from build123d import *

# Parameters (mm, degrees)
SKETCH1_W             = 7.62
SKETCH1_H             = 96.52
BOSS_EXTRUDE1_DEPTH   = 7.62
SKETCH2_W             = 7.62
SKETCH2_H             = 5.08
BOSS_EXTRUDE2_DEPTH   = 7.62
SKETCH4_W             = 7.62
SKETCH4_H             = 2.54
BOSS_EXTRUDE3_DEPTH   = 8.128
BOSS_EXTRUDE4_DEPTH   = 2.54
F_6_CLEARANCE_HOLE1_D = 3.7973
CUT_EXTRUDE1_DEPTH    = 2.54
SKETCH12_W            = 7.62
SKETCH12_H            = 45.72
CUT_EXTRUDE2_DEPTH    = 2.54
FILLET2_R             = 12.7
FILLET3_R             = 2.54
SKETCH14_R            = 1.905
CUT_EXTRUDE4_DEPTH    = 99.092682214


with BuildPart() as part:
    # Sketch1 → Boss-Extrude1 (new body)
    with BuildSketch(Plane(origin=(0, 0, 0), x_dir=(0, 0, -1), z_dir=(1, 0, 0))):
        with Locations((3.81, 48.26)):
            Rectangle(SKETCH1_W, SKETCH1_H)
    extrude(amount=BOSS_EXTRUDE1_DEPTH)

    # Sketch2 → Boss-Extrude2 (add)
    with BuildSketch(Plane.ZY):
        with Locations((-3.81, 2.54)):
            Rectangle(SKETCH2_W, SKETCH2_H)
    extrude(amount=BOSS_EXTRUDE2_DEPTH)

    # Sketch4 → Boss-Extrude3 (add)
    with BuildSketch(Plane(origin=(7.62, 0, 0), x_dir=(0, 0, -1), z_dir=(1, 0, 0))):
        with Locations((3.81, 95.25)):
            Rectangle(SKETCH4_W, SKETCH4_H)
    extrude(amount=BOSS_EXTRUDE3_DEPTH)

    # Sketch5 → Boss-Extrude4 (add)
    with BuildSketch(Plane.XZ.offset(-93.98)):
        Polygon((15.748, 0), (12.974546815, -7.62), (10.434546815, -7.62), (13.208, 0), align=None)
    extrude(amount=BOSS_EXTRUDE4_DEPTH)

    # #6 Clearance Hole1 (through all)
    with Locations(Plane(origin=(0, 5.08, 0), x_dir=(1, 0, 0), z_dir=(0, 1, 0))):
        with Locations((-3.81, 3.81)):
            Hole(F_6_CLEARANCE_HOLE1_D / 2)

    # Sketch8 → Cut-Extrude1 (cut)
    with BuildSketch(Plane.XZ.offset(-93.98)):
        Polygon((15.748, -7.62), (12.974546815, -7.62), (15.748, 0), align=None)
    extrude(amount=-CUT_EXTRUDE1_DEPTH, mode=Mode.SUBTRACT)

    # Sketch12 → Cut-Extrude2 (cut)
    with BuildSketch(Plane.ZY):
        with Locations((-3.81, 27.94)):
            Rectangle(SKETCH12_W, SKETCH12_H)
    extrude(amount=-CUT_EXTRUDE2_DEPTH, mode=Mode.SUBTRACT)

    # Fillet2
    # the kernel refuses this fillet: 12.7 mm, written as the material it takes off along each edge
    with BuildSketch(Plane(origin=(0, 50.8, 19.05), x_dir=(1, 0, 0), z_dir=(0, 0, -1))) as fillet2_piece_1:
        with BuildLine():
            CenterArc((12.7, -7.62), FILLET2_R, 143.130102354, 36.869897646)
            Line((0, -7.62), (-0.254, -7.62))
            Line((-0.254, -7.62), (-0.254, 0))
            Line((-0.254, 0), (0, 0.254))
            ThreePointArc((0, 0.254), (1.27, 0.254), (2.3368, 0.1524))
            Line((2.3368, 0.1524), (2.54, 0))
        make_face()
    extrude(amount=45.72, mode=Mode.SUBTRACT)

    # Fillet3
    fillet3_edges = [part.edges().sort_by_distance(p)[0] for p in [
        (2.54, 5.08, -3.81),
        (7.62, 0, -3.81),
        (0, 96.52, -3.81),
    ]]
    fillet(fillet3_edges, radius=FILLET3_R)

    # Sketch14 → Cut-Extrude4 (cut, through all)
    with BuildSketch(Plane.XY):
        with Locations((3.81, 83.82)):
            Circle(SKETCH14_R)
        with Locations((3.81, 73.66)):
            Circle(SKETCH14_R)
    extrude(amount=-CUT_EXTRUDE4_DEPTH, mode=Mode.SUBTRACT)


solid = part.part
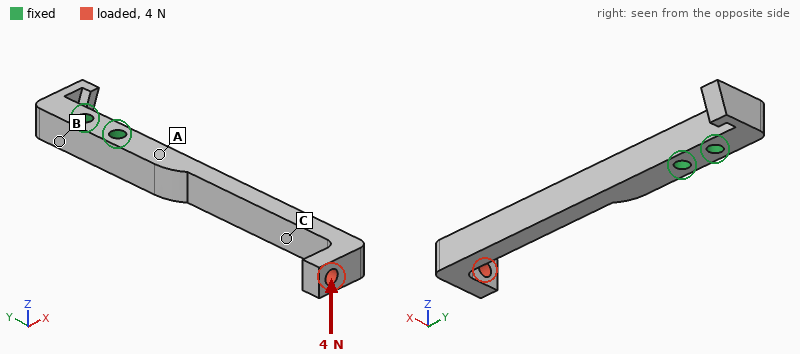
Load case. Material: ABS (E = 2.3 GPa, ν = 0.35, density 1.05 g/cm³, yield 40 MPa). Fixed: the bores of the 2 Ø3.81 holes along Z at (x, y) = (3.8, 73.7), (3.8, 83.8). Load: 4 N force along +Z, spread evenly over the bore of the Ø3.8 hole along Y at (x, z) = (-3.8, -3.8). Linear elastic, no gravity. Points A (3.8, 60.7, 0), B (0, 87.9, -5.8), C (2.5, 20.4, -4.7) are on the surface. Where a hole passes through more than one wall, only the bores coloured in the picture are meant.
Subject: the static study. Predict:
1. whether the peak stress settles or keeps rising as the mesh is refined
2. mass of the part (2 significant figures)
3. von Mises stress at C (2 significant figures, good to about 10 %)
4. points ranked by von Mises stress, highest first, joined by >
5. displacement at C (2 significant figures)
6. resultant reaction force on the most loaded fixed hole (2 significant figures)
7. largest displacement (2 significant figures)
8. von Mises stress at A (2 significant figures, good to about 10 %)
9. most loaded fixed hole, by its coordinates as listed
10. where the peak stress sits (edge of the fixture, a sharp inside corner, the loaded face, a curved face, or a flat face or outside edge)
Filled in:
keeps rising
5.2 g
1.6 MPa
A > C > B
0.55 mm
5.4 N
1.1 mm
3.2 MPa
(3.8, 73.7)
edge of the fixture
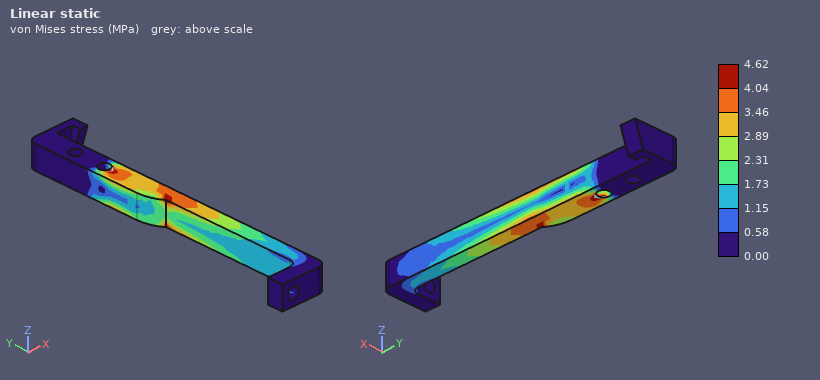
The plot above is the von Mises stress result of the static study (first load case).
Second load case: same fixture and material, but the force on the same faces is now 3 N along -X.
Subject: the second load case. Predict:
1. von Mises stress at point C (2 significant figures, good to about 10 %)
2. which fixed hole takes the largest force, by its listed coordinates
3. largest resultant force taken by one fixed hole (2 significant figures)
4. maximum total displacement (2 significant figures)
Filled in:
1.6 MPa
(3.8, 73.7)
7.2 N
1.2 mm
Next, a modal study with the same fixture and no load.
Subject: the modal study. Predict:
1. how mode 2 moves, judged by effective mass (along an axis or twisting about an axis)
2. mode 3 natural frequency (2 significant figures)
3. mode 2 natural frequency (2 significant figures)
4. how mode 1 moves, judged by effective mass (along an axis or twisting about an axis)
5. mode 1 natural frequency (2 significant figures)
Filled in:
along Z
1400 Hz
320 Hz
along X
260 Hz
